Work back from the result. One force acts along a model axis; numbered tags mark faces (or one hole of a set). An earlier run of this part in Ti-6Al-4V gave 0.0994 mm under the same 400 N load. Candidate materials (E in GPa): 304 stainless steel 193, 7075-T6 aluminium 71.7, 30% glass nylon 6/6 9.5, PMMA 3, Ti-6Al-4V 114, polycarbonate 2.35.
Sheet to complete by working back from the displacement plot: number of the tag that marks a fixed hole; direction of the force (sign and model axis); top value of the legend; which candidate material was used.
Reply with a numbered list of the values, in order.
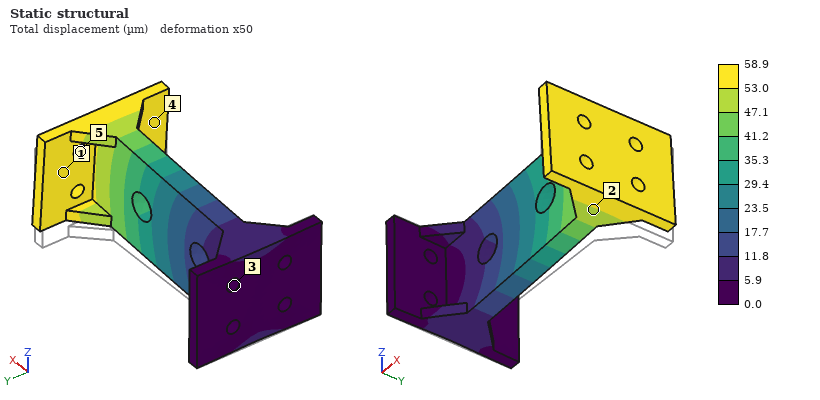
1. 3
2. +Z
3. 58.9 µm
4. 304 stainless steel
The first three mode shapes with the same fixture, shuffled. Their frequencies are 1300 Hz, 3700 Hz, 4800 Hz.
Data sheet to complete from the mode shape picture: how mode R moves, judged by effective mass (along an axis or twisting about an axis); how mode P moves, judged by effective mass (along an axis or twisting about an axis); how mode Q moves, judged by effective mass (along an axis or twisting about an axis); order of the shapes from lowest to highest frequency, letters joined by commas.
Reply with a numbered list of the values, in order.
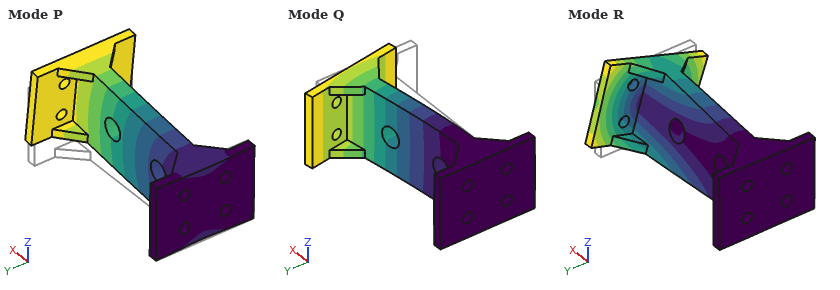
1. twisting about X
2. along Z
3. along Y
4. Q, P, R
